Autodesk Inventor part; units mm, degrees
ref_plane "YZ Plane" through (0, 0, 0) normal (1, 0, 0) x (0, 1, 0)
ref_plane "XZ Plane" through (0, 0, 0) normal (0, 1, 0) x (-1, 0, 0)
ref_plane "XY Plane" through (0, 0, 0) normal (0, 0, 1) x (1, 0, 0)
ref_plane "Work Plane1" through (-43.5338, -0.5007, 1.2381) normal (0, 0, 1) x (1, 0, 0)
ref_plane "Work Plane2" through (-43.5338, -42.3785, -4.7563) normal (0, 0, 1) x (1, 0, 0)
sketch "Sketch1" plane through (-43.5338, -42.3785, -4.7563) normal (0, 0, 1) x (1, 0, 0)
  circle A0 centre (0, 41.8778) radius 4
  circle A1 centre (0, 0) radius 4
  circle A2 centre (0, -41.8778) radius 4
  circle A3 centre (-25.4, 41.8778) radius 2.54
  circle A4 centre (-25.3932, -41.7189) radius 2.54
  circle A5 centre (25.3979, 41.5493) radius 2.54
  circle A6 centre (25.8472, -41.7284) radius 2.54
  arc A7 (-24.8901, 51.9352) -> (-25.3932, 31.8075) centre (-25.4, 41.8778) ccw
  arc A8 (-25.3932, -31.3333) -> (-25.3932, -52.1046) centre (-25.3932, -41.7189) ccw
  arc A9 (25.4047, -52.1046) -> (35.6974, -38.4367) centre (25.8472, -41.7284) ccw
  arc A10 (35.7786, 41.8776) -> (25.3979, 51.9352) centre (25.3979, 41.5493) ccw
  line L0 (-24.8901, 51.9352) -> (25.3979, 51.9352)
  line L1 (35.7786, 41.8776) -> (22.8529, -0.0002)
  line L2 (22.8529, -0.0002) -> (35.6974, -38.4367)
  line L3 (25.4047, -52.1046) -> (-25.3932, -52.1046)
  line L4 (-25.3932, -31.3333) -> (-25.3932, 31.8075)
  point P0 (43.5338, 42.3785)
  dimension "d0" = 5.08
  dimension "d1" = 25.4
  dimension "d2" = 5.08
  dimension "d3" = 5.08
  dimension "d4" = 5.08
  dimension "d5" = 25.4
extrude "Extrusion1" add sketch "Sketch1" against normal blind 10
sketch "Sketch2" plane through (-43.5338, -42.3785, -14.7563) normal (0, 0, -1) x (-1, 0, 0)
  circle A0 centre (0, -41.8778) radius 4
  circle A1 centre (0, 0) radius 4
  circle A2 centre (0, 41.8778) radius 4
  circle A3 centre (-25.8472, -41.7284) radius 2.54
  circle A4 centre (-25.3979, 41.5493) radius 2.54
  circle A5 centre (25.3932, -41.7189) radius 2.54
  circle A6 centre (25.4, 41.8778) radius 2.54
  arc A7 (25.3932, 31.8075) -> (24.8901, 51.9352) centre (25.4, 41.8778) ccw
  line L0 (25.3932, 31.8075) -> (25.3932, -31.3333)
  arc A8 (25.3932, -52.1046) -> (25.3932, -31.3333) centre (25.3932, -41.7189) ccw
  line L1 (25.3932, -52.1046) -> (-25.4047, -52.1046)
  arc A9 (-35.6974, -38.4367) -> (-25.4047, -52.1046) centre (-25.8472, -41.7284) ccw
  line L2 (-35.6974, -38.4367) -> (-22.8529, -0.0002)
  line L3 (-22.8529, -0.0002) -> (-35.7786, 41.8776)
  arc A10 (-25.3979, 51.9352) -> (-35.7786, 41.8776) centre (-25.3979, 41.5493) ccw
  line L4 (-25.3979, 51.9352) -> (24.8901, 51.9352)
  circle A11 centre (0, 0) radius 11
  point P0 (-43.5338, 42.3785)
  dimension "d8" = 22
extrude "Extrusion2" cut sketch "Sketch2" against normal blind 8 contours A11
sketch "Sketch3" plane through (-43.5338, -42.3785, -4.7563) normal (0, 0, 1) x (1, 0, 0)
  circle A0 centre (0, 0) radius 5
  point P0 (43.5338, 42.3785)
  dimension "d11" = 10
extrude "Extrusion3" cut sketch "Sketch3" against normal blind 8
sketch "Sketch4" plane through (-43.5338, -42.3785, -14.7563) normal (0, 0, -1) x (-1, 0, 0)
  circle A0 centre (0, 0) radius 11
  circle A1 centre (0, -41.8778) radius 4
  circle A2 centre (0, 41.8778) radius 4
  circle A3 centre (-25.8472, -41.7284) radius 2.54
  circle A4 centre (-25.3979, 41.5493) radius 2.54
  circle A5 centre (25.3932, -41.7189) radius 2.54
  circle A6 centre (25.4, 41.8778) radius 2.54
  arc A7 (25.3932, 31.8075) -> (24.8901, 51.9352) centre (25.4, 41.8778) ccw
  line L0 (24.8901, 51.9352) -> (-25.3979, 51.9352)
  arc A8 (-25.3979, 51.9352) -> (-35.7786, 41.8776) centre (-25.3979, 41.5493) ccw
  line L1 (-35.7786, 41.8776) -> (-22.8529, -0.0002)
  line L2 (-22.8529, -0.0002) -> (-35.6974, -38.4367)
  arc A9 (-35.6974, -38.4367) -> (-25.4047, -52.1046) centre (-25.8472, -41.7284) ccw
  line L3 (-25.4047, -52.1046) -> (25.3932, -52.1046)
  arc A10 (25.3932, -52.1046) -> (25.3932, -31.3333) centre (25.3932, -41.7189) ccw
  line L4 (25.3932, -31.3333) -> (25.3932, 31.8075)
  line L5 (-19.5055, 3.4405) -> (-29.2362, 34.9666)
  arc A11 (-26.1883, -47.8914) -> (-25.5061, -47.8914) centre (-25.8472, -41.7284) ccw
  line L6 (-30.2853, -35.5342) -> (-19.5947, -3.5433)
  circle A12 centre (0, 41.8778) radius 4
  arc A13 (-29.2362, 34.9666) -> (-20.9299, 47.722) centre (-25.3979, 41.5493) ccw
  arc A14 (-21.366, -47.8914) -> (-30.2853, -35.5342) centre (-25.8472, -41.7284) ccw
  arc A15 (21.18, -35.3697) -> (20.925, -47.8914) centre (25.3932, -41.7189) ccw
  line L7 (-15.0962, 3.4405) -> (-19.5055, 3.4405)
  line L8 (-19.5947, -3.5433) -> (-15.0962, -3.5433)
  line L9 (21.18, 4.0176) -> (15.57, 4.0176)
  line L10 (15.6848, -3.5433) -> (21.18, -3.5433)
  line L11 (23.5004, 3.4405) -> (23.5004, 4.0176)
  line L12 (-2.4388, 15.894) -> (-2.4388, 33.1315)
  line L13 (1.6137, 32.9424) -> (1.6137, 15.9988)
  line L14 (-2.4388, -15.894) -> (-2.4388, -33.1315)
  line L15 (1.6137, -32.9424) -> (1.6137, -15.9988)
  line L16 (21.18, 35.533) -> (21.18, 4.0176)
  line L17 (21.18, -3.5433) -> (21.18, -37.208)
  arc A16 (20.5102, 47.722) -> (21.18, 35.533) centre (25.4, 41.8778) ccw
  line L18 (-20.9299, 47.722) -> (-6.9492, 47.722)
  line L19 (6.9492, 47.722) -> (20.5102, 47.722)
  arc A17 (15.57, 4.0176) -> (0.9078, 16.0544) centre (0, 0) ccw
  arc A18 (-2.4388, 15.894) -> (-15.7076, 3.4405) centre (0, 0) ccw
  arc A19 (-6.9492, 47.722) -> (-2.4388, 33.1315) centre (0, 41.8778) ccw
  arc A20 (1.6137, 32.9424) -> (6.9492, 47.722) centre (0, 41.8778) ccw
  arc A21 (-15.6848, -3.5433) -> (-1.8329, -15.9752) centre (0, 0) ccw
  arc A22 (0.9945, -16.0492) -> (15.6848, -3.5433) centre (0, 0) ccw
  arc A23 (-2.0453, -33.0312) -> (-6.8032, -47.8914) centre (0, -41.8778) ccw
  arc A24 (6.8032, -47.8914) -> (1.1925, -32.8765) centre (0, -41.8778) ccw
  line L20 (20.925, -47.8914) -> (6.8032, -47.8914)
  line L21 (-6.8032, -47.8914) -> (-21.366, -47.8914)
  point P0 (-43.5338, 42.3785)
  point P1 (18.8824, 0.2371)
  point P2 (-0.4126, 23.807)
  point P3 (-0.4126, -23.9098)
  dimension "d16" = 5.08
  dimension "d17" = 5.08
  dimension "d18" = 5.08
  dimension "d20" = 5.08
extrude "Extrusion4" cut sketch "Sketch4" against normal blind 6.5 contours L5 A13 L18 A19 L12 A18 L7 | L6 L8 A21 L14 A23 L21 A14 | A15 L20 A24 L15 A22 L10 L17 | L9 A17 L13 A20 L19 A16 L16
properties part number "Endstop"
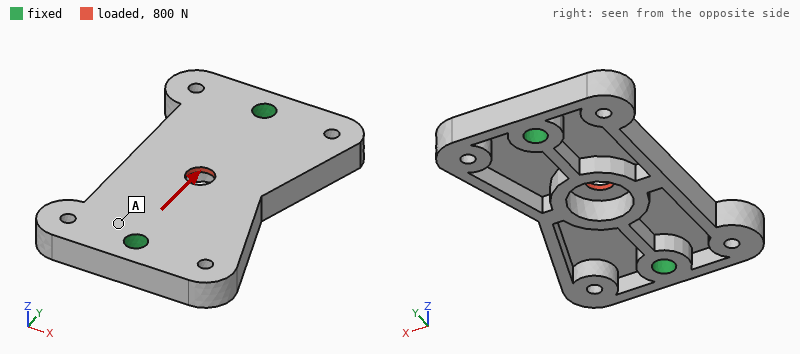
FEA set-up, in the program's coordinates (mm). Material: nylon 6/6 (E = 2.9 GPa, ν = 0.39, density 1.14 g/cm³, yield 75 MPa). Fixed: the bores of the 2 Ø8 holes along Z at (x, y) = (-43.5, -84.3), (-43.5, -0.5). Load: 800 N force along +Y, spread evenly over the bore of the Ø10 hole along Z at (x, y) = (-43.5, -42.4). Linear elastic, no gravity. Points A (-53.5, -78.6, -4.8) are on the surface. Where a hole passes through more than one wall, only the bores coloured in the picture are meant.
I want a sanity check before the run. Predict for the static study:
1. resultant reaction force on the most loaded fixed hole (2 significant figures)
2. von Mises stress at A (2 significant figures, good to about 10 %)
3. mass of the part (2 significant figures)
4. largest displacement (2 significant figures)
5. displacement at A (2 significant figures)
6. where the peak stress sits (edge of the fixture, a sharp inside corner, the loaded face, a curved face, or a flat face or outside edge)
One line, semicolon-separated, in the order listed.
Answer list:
400 N; 1.6 MPa; 44 g; 73 µm; 12 µm; the loaded face
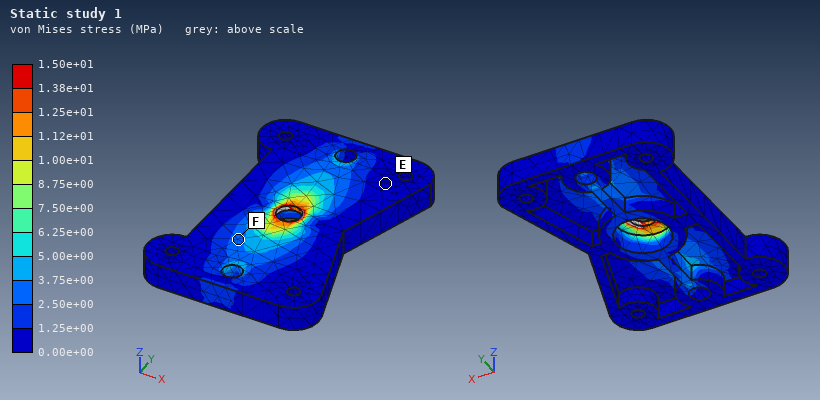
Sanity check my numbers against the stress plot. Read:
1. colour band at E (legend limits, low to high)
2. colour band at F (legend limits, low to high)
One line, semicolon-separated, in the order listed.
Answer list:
0.00e+00 to 1.25e+00 MPa; 2.50e+00 to 3.75e+00 MPa
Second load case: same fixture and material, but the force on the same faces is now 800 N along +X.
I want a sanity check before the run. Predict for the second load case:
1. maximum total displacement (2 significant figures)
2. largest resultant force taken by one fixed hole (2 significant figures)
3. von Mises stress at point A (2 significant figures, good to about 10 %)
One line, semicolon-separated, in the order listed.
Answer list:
0.16 mm; 400 N; 3.7 MPa
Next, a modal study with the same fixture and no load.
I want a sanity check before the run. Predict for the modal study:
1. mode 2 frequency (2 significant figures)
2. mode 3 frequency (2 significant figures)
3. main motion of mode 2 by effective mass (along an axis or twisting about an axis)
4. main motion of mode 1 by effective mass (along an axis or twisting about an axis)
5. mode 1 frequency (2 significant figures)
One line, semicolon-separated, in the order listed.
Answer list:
1200 Hz; 1600 Hz; along Z; twisting about Y; 1000 Hz
